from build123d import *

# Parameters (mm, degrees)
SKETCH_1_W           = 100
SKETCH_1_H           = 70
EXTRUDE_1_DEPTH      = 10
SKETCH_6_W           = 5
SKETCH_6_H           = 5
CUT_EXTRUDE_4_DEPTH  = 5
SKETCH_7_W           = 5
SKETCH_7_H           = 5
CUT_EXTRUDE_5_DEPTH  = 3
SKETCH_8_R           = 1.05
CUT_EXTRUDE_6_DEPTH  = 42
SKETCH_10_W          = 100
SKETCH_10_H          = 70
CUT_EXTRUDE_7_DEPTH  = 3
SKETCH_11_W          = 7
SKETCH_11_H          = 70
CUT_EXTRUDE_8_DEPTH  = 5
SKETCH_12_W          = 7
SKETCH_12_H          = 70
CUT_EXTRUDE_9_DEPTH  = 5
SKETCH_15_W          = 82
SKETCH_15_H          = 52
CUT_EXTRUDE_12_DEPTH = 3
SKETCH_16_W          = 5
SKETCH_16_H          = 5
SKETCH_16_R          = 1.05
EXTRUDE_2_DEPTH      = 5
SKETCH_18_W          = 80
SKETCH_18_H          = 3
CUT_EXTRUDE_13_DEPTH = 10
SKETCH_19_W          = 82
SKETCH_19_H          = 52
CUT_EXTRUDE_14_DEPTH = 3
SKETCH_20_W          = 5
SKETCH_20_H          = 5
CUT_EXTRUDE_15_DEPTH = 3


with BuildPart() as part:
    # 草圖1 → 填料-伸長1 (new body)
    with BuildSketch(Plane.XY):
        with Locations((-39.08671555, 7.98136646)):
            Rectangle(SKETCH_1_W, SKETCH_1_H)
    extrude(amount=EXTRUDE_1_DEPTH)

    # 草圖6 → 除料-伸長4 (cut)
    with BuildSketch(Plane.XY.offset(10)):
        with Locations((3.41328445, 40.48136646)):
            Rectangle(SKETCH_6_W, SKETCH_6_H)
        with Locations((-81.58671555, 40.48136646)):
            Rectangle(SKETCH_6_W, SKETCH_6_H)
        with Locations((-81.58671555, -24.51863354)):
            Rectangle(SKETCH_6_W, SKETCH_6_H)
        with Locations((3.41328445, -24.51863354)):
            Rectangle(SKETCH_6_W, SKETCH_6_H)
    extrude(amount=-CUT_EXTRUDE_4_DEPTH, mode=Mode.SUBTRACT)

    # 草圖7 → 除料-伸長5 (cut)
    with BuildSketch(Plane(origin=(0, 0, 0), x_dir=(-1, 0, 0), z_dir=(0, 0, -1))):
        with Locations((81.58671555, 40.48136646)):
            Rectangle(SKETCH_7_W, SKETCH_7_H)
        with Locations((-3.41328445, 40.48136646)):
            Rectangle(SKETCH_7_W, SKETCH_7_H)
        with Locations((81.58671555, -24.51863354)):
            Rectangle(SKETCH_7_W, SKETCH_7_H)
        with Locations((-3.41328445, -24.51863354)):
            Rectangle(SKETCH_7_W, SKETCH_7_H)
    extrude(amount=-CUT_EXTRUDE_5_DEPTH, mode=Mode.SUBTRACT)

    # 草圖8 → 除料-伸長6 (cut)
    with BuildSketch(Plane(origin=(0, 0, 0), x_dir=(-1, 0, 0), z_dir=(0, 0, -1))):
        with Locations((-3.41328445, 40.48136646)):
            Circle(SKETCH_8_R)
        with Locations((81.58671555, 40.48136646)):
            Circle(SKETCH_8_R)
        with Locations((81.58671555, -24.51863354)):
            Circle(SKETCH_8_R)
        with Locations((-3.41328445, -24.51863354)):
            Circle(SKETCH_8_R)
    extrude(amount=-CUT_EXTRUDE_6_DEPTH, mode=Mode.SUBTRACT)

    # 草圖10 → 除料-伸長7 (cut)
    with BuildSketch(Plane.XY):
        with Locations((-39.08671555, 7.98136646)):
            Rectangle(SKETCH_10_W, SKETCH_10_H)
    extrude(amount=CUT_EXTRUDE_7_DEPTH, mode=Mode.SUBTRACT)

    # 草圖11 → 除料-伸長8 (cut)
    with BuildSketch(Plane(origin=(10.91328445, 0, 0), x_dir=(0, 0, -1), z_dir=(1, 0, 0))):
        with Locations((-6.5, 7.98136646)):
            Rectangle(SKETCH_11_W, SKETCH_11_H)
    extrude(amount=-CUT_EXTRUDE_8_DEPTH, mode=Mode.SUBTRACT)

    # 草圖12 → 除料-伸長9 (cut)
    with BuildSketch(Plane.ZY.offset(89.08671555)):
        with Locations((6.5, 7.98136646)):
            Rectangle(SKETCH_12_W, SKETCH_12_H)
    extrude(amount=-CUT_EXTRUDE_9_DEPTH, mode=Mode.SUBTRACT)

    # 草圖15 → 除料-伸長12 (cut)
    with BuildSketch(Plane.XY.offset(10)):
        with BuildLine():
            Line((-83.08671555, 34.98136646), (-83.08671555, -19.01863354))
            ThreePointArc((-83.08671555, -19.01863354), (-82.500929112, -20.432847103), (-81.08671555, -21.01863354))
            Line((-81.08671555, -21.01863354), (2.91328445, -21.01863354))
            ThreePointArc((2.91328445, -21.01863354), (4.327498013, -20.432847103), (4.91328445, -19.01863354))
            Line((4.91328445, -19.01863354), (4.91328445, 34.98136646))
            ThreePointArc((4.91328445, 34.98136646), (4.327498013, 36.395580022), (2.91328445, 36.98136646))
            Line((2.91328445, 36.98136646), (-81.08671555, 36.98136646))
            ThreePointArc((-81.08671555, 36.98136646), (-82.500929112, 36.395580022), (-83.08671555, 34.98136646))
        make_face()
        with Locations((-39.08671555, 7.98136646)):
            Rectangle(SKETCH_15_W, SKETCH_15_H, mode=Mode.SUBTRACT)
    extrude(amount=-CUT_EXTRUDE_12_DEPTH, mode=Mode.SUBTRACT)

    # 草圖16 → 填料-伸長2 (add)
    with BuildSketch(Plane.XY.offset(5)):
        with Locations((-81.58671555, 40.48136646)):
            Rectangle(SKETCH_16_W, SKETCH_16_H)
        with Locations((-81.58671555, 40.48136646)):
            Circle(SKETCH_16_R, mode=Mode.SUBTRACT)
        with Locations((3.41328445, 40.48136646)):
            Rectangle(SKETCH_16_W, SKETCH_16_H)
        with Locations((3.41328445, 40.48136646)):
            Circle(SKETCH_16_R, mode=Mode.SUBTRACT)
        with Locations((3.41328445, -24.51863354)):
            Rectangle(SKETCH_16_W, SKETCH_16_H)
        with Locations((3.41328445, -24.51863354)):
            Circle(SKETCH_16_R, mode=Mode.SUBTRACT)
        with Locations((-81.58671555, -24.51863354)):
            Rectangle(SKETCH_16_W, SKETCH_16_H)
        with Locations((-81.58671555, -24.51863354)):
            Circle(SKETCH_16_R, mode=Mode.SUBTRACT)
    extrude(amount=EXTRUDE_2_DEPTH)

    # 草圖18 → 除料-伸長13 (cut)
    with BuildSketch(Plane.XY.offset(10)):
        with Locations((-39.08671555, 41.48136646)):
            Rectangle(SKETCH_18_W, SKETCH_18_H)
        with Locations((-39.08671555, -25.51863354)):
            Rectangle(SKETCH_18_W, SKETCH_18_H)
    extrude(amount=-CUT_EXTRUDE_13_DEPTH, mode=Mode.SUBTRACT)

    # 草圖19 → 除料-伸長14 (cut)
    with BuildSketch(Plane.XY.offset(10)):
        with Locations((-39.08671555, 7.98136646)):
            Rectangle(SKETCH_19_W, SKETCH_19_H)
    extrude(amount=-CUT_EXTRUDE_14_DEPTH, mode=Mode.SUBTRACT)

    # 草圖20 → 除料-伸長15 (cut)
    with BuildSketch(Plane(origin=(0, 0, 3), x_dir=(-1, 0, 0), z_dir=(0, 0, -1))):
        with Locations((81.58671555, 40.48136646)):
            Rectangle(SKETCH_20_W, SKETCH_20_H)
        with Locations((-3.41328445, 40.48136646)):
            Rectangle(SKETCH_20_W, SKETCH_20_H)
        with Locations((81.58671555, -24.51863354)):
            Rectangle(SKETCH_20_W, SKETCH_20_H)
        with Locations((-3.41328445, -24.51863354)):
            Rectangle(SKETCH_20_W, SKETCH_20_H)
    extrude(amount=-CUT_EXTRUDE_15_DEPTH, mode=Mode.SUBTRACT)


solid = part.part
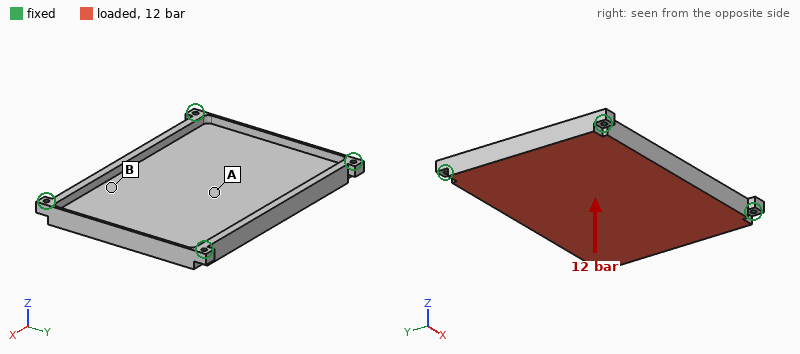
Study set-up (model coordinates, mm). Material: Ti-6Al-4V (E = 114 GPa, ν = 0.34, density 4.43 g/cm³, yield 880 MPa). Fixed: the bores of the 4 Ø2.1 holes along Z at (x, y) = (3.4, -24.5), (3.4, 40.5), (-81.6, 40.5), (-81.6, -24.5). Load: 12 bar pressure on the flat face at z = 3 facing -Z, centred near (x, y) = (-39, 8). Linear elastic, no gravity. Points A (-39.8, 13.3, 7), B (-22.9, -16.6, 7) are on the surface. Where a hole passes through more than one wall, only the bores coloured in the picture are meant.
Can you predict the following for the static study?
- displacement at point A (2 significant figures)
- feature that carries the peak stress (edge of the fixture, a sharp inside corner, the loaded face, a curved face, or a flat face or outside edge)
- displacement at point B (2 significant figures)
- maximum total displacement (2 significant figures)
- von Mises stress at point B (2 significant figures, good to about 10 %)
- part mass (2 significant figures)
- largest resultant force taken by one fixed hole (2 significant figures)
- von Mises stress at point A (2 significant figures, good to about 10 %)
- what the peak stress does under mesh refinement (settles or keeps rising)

0.44 mm
edge of the fixture
0.29 mm
0.44 mm
51 MPa
110 g
4.5 kN
120 MPa
keeps rising
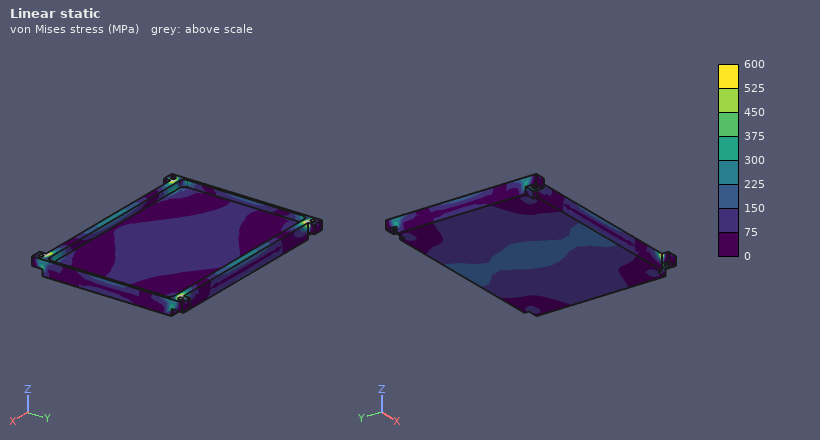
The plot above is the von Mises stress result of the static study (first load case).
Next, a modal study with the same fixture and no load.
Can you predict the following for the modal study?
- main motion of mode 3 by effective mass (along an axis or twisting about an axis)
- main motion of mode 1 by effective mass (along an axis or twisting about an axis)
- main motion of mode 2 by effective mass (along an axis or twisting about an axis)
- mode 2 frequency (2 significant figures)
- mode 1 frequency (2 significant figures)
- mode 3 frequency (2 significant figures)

twisting about Y
along Z
twisting about X
3700 Hz
2300 Hz
4600 Hz
